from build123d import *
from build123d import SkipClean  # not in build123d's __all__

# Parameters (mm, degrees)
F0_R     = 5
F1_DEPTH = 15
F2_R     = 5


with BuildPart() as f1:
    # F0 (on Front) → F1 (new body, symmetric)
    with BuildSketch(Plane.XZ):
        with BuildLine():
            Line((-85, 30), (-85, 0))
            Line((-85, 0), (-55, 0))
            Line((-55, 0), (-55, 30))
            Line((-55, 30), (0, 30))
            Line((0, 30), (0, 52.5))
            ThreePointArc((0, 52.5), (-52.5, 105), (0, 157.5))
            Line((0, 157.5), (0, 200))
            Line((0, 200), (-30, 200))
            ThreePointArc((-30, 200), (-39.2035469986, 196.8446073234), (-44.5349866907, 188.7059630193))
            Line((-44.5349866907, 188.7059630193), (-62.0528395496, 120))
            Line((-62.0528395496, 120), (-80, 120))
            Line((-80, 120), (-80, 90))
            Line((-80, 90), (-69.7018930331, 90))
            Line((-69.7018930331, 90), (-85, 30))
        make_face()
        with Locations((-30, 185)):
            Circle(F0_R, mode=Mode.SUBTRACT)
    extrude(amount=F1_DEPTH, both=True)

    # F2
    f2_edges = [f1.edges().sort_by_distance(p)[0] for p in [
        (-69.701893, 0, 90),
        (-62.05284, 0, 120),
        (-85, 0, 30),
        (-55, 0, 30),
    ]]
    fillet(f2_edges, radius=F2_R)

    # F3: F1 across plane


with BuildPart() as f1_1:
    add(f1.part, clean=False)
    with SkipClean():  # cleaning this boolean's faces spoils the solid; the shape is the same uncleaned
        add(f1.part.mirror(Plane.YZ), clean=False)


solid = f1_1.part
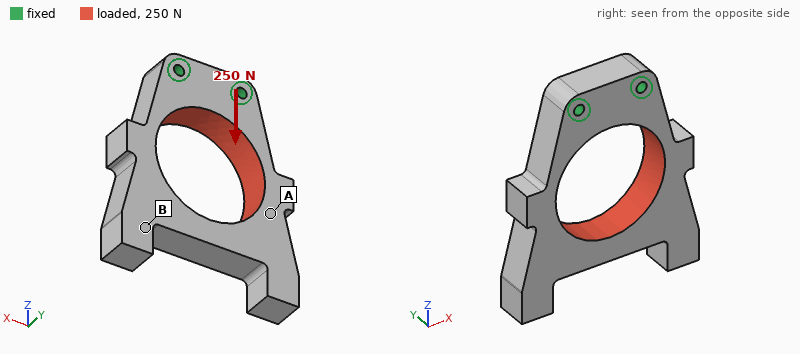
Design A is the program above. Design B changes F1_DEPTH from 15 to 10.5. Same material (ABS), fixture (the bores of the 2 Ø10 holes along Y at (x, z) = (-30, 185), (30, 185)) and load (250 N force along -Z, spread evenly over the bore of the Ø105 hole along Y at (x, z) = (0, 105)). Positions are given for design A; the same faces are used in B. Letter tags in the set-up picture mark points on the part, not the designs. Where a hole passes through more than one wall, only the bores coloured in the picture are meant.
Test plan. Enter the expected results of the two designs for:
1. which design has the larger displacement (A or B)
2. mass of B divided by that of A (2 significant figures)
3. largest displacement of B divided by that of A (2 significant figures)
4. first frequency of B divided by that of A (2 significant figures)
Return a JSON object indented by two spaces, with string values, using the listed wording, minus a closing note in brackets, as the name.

{
  "which design has the larger displacement": "B",
  "mass of B divided by that of A": "0.70",
  "largest displacement of B divided by that of A": "1.4",
  "first frequency of B divided by that of A": "0.73"
}
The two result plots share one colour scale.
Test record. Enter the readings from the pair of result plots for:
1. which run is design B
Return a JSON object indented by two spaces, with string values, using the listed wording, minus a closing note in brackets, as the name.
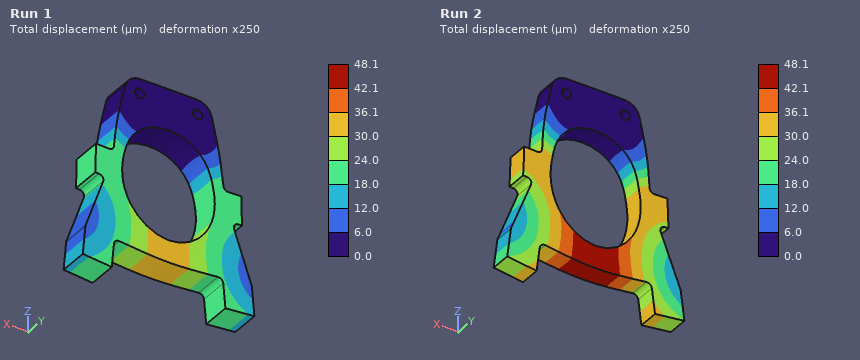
{
  "which run is design B": "Run 2"
}
